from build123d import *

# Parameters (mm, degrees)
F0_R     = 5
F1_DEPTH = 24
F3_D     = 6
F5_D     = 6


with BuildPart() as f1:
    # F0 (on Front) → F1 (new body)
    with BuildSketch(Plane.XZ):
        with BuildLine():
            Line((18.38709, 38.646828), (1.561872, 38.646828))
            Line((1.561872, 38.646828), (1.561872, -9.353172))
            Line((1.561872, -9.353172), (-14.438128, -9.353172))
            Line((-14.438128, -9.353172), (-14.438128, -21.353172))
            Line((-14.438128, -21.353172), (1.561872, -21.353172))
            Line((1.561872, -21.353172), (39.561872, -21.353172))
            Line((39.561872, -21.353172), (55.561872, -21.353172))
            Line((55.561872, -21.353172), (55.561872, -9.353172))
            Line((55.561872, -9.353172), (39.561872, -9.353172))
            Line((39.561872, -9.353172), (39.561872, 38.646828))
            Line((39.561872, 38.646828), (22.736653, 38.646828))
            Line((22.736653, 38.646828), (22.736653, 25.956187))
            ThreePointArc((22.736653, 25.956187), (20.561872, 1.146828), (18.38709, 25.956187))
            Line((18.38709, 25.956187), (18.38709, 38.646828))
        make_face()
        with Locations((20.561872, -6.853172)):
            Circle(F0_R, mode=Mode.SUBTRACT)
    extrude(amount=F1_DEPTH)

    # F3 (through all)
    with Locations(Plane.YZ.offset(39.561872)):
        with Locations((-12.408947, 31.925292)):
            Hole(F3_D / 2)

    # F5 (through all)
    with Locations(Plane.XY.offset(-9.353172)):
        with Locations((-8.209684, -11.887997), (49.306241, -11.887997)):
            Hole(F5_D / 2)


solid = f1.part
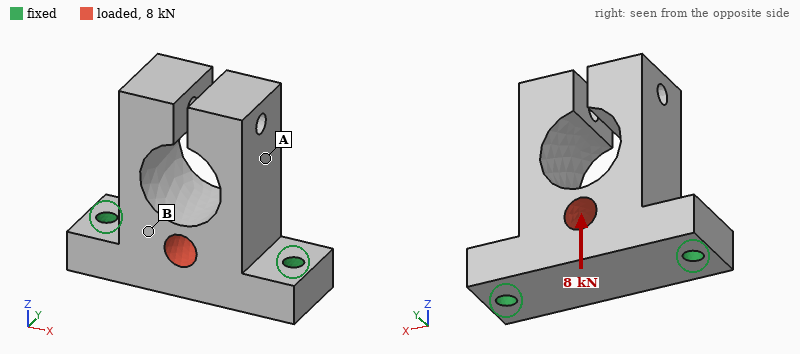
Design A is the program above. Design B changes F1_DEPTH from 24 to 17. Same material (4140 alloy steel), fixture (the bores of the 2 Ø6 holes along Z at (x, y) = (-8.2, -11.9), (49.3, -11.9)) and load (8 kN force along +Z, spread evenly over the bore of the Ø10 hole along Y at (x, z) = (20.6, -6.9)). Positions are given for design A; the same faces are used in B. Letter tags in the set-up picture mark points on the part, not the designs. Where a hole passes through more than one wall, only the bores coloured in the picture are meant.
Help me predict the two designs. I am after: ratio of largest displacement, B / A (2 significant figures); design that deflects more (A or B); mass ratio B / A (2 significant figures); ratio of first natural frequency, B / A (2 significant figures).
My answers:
1.7
B
0.70
0.90
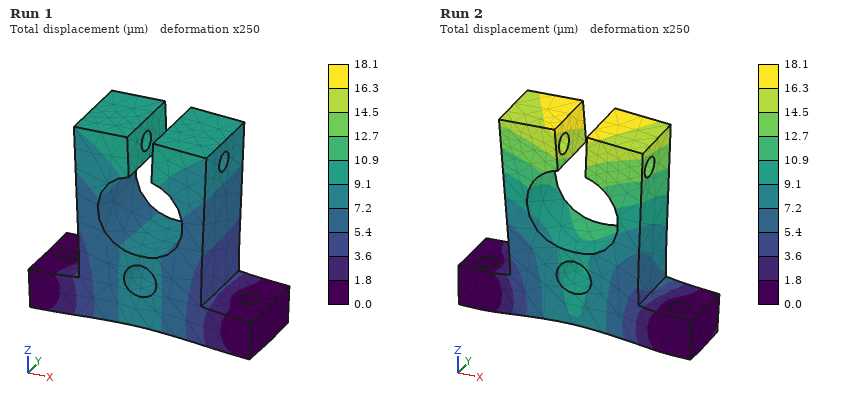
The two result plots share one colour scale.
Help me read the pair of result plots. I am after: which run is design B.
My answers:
Run 2
